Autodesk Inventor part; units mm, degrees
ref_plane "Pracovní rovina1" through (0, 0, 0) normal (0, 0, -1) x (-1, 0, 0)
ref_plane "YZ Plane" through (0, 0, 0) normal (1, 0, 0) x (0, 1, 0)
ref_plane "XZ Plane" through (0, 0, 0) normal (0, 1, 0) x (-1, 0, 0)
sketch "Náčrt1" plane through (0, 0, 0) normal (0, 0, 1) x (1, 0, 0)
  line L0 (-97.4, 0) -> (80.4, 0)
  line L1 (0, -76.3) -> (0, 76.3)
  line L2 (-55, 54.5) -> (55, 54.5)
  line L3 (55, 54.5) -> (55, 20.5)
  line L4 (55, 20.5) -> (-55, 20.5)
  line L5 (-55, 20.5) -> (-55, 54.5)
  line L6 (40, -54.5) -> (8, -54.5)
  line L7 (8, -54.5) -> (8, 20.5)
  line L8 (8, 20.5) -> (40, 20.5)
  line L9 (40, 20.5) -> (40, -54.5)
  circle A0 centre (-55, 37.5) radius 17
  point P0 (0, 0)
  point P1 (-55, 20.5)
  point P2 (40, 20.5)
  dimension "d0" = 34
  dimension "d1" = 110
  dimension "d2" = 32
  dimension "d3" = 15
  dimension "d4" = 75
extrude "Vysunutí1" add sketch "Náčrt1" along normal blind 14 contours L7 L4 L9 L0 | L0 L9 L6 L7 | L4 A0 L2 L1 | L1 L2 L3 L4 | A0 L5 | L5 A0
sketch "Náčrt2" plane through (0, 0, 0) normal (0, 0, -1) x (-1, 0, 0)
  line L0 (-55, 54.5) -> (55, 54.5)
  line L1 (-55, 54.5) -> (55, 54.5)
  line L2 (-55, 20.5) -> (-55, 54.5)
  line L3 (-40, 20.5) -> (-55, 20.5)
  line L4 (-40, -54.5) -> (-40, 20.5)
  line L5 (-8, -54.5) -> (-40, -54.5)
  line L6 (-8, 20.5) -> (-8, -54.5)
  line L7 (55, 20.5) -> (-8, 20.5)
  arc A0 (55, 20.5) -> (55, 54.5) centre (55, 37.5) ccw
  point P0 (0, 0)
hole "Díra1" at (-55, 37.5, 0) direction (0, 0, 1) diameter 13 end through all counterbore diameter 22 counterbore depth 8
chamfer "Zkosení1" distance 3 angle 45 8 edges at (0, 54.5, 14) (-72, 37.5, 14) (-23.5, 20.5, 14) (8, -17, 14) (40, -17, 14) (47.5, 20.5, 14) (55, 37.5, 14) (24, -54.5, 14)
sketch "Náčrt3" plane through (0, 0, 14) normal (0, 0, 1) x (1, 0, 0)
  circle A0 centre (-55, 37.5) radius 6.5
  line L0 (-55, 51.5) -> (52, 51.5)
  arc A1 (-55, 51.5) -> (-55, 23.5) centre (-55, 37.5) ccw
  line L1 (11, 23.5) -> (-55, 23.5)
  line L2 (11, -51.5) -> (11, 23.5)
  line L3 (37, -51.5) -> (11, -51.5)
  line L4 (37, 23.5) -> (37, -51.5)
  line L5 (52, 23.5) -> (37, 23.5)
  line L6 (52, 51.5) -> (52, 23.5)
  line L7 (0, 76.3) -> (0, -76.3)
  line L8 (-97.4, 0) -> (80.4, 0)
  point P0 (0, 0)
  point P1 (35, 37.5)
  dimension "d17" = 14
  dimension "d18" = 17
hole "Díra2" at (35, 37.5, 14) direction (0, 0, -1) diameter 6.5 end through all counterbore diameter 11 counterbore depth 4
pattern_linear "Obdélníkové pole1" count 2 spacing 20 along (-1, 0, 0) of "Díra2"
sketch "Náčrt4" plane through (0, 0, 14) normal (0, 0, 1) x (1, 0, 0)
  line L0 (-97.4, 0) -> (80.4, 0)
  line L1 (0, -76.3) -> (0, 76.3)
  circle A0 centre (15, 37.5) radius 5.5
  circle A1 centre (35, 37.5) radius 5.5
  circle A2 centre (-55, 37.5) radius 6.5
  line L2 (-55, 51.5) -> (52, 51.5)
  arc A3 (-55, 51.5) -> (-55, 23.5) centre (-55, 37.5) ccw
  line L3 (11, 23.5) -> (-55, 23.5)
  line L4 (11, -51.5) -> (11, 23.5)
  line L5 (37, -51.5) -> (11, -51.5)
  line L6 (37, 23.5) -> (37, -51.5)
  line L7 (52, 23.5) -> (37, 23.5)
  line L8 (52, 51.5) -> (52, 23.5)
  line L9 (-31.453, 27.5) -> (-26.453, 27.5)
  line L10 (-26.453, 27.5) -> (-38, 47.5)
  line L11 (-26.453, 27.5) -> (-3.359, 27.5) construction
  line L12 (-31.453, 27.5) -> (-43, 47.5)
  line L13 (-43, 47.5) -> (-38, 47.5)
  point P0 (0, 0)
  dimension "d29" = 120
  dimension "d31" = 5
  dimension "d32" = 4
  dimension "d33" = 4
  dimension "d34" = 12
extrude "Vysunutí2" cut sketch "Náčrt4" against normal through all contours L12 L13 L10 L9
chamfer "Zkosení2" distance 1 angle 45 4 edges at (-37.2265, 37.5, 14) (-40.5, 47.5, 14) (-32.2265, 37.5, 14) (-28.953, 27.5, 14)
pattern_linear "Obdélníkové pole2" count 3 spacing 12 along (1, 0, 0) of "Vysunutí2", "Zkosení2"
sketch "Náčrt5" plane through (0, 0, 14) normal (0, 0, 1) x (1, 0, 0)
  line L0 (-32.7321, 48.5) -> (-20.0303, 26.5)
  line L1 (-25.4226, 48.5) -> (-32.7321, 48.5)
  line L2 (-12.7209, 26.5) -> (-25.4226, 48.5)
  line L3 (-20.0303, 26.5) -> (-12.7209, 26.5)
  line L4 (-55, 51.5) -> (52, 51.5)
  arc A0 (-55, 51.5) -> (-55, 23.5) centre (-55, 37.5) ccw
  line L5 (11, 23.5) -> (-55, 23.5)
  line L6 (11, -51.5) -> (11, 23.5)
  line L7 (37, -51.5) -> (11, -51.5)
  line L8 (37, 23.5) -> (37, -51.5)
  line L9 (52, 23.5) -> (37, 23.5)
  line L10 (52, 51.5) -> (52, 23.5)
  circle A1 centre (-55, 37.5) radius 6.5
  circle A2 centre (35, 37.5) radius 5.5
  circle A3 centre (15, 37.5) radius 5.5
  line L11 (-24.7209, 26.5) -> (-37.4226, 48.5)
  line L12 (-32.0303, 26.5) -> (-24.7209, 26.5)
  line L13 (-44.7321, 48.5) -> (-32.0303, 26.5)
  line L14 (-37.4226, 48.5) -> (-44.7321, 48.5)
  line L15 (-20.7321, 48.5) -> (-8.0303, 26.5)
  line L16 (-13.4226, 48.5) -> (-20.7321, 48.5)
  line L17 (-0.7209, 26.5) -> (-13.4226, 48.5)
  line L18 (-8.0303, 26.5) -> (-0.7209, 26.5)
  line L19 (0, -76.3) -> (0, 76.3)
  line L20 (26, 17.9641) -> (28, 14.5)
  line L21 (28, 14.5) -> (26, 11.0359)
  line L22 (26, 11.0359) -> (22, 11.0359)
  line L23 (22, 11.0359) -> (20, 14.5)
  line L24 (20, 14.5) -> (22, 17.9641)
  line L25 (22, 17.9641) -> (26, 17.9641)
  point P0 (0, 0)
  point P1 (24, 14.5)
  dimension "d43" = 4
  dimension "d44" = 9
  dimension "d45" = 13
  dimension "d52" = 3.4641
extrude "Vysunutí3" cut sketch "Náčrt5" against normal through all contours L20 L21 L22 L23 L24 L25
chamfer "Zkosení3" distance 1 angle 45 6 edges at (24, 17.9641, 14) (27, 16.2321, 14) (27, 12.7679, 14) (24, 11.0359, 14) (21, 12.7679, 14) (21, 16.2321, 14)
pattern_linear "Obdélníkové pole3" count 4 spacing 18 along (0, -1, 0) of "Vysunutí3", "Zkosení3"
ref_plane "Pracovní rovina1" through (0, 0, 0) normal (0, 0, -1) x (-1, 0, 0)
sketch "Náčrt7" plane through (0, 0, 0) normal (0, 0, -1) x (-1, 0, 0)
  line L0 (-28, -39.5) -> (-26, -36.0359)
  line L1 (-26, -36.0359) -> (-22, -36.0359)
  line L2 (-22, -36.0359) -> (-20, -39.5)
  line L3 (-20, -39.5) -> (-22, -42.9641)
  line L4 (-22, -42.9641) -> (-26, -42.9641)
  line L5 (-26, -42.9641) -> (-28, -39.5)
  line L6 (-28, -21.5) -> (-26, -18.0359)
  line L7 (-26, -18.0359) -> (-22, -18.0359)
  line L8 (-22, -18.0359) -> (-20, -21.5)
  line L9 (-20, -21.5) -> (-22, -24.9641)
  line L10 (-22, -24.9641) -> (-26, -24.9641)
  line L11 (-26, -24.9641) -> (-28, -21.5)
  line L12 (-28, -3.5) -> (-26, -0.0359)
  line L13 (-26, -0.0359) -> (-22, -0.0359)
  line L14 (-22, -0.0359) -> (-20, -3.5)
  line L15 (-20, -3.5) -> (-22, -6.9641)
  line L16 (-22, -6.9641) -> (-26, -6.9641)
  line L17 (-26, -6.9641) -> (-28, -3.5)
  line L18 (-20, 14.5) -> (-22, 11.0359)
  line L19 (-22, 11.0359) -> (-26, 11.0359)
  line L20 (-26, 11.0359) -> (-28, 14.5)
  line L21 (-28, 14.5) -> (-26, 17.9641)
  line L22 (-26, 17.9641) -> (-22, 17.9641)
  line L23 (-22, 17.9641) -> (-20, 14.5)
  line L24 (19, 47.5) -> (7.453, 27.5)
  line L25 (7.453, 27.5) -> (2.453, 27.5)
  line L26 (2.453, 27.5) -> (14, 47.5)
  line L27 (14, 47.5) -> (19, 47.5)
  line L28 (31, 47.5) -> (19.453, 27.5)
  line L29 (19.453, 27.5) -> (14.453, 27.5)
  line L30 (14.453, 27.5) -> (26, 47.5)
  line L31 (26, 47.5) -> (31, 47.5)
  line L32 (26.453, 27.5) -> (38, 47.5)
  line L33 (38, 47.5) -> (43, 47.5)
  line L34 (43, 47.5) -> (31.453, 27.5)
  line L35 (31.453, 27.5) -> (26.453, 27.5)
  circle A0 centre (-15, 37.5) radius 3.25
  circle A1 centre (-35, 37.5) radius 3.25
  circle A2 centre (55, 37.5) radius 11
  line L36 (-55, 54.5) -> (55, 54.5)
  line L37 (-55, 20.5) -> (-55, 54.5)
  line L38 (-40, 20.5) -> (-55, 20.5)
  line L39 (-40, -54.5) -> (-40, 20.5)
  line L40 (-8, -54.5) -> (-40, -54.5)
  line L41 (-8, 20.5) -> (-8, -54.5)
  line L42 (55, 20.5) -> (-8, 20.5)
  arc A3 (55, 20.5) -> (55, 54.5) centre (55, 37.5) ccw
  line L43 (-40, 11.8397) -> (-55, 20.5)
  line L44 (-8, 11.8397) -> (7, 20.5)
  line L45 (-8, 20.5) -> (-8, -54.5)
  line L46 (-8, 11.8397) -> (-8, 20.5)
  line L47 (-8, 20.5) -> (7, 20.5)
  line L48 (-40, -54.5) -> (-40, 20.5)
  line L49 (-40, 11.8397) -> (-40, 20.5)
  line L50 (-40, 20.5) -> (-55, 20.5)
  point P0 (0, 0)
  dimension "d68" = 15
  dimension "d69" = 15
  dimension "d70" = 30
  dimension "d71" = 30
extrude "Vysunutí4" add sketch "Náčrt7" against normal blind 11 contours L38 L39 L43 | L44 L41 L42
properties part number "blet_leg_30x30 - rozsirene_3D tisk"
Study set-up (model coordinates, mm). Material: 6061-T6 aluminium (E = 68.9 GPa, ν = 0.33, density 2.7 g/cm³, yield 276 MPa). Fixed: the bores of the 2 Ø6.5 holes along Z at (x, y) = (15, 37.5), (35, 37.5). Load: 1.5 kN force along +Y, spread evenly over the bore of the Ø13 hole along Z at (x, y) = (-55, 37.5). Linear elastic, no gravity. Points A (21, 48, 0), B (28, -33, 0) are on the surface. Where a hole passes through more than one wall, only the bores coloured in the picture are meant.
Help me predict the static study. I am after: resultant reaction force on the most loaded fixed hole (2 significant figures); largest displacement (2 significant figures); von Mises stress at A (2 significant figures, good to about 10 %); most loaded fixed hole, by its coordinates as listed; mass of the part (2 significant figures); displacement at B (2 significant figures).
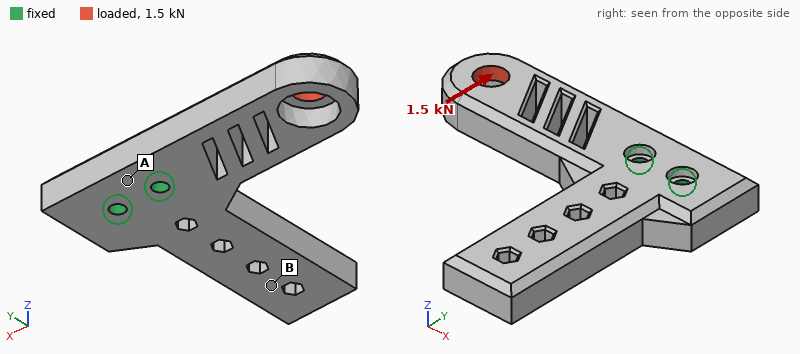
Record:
5.3 kN
0.17 mm
24 MPa
(15, 37.5)
220 g
0.029 mm
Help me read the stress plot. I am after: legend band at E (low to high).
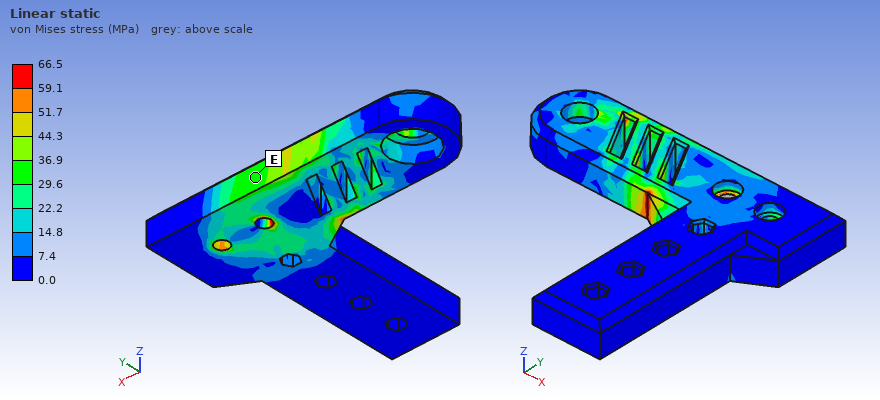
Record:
29.6 to 36.9 MPa
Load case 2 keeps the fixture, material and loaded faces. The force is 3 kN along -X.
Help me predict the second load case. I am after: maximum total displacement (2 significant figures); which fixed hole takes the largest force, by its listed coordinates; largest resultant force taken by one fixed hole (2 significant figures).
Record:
0.18 mm
(15, 37.5)
2.0 kN
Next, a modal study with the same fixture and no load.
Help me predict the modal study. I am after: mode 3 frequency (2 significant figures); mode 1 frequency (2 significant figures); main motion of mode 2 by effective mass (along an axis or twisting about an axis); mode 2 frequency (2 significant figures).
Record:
2700 Hz
1300 Hz
along Z
1500 Hz
